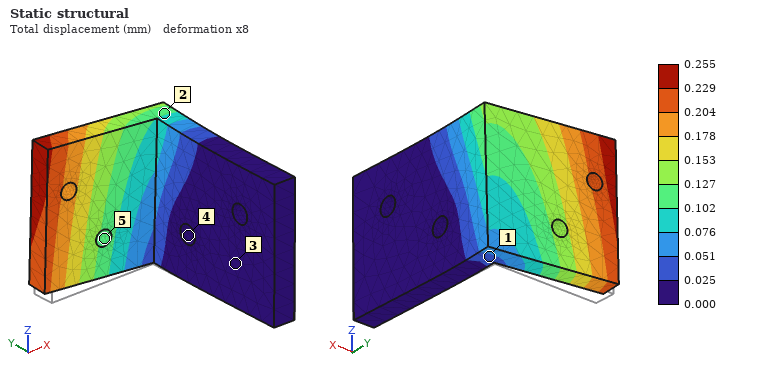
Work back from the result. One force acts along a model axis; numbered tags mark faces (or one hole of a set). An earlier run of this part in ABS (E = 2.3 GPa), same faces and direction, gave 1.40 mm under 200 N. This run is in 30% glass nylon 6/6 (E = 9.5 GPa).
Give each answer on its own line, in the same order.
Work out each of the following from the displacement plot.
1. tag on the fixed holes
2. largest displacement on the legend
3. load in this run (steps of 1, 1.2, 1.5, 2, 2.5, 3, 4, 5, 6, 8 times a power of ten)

4
0.255 mm
150 N
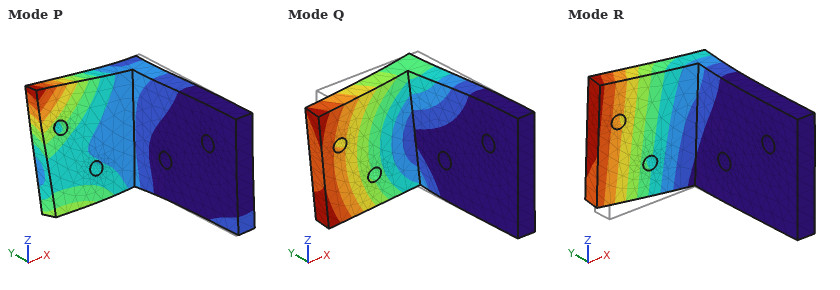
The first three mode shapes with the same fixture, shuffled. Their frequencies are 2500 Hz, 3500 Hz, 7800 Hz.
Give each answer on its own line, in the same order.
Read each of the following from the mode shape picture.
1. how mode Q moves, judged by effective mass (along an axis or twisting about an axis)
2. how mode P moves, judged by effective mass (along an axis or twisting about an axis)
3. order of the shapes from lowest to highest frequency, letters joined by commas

along Z
along X
R, Q, P
